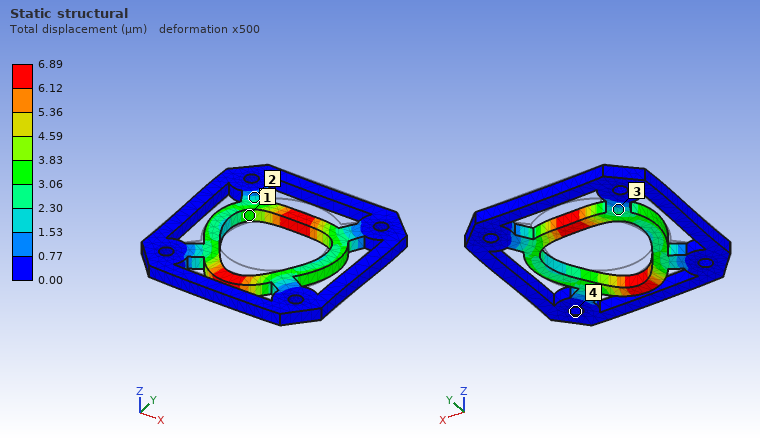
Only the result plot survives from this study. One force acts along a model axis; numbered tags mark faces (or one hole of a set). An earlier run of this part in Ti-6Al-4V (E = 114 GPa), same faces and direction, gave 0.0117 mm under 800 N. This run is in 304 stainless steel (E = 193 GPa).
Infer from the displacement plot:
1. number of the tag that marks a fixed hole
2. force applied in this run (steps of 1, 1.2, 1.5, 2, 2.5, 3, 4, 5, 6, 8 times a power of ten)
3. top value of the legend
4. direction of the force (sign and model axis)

4
800 N
6.89 µm
-Y
